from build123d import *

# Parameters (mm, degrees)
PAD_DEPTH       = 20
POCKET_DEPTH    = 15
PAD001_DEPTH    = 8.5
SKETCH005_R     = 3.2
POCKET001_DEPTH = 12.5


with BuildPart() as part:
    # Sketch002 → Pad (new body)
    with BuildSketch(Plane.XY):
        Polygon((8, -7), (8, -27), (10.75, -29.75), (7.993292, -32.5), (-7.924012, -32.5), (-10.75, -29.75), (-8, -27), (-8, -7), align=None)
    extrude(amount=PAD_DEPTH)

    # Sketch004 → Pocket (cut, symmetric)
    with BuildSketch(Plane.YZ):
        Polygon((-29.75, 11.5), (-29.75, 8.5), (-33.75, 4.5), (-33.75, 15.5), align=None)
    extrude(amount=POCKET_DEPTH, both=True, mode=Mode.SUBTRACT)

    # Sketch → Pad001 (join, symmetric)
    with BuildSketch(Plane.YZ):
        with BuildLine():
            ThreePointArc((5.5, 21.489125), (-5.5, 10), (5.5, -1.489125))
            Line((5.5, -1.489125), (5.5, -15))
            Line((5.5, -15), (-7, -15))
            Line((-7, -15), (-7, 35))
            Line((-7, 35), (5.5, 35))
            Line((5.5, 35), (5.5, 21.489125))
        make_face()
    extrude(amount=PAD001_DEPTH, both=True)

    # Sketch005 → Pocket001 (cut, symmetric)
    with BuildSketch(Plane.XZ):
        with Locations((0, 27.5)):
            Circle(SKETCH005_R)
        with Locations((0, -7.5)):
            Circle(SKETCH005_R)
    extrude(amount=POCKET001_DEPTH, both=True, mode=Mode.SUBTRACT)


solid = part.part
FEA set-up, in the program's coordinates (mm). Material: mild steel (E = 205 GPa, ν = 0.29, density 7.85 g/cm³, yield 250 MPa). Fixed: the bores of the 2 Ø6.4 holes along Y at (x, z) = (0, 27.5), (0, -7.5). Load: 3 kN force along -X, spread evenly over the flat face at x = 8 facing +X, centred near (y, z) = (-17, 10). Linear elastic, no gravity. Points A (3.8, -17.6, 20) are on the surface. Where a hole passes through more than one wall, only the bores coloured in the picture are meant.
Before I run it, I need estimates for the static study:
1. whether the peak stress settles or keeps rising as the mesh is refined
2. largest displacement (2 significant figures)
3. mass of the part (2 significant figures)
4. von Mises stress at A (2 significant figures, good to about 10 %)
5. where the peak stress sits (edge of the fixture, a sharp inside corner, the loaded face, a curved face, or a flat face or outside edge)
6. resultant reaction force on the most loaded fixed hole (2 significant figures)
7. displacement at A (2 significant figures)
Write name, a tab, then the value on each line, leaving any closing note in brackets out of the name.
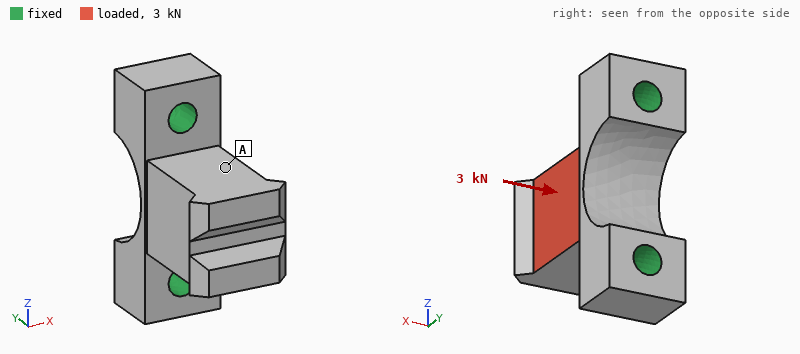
whether the peak stress settles or keeps rising as the mesh is refined	keeps rising
largest displacement	31 µm
mass of the part	120 g
von Mises stress at A	17 MPa
where the peak stress sits	edge of the fixture
resultant reaction force on the most loaded fixed hole	1.5 kN
displacement at A	16 µm
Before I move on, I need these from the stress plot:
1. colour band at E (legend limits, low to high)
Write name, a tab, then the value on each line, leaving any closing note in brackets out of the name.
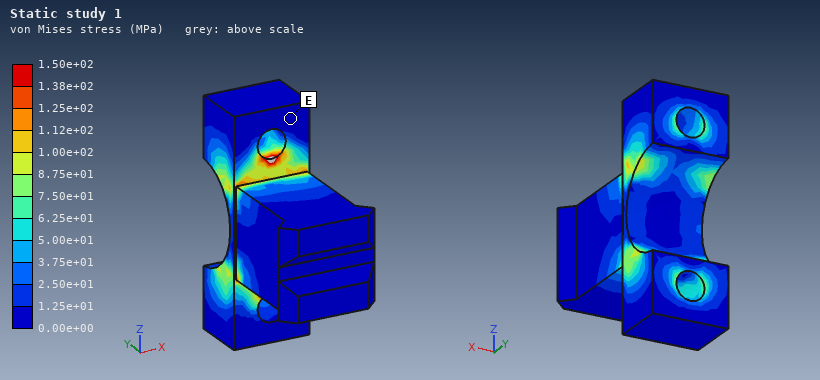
colour band at E	0.00e+00 to 1.25e+01 MPa
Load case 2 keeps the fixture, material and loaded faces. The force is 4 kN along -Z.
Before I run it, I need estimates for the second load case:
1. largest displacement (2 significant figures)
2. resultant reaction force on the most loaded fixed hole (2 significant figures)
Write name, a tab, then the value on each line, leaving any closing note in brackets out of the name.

largest displacement	15 µm
resultant reaction force on the most loaded fixed hole	3.2 kN
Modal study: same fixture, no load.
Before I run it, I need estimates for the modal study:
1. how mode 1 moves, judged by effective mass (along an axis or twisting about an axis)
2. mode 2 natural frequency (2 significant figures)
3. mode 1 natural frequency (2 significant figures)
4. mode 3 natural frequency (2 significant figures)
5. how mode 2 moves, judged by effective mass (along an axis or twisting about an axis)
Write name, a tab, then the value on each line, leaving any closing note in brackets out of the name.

how mode 1 moves, judged by effective mass	along X
mode 2 natural frequency	12 kHz
mode 1 natural frequency	6700 Hz
mode 3 natural frequency	22 kHz
how mode 2 moves, judged by effective mass	along Z
